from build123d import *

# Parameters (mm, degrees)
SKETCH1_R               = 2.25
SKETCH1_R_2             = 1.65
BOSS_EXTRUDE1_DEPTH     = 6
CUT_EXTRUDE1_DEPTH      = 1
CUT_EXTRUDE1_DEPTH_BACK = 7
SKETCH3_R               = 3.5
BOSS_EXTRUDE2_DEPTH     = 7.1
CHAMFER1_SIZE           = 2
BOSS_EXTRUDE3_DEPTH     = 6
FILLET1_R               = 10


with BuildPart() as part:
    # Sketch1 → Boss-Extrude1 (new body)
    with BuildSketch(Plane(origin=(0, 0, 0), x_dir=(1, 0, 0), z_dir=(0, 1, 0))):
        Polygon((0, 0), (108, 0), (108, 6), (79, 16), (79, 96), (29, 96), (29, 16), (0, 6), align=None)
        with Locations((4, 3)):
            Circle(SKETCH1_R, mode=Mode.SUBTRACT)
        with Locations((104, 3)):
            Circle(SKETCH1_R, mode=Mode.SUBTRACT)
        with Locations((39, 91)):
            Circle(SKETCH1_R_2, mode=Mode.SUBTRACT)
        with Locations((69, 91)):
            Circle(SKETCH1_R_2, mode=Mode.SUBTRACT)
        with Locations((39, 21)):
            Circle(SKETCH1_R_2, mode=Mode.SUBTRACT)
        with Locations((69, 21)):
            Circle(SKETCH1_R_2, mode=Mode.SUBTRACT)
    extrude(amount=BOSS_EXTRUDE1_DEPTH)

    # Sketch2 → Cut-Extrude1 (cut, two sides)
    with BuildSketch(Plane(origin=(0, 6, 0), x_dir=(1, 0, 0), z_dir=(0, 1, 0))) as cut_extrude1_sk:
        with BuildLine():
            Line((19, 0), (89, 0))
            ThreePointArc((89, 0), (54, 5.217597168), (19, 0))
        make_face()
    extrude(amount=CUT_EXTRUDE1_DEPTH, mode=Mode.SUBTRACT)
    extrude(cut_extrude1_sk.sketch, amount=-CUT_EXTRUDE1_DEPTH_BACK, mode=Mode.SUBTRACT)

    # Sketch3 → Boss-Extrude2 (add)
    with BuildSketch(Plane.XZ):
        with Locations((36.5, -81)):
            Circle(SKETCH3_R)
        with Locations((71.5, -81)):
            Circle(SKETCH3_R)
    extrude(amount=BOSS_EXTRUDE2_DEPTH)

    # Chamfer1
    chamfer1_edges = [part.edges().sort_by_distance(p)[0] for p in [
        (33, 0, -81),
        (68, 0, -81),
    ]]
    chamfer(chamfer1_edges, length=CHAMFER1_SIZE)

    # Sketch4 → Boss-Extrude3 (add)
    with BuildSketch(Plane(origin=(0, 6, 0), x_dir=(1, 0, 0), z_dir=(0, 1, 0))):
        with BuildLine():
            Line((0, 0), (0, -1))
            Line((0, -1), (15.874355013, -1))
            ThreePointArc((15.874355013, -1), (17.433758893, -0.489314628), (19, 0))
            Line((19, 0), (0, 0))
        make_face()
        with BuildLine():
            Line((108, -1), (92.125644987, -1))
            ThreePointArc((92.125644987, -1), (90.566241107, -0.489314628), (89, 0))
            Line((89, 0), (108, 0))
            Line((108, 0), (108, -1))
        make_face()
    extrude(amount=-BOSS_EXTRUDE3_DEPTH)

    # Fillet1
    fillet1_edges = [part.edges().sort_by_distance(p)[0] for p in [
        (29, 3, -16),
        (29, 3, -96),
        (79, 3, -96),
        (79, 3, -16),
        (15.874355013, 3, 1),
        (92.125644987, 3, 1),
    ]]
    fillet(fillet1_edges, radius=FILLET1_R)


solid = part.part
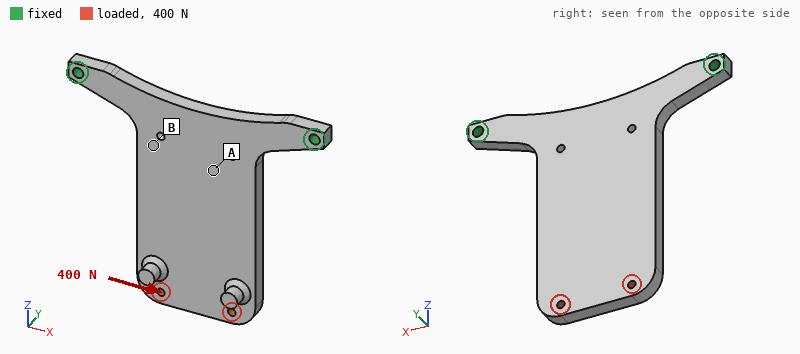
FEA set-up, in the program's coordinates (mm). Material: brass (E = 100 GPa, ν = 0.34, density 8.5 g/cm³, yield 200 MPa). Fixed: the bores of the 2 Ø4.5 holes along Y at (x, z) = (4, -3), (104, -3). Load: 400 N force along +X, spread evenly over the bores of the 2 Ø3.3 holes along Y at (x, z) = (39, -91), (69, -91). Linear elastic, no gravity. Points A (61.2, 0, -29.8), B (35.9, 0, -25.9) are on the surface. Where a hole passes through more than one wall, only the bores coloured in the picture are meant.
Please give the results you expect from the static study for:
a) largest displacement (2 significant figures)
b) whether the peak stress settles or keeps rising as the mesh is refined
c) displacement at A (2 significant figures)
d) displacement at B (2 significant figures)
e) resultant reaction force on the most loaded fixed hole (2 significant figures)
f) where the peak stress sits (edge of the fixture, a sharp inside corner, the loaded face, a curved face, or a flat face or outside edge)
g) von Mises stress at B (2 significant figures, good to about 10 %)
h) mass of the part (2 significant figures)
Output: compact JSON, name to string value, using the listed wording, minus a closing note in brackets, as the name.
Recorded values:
{"largest displacement": "50 µm", "whether the peak stress settles or keeps rising as the mesh is refined": "keeps rising", "displacement at A": "8.2 µm", "displacement at B": "10 µm", "resultant reaction force on the most loaded fixed hole": "460 N", "where the peak stress sits": "edge of the fixture", "von Mises stress at B": "8.6 MPa", "mass of the part": "270 g"}
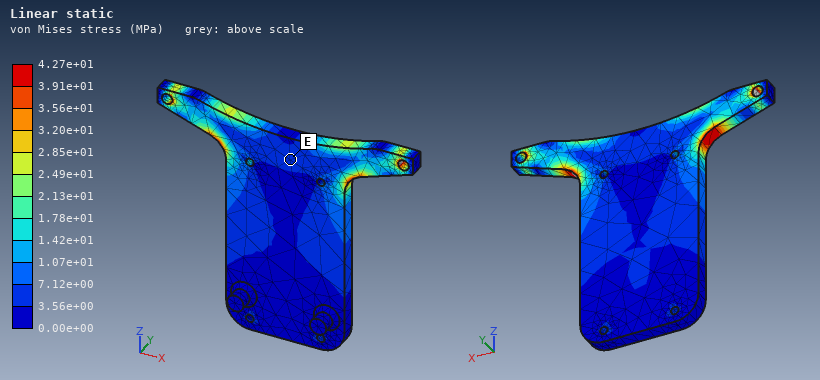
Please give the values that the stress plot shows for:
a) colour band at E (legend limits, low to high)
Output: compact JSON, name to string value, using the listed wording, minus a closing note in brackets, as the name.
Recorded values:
{"colour band at E": "3.56e+00 to 7.12e+00 MPa"}
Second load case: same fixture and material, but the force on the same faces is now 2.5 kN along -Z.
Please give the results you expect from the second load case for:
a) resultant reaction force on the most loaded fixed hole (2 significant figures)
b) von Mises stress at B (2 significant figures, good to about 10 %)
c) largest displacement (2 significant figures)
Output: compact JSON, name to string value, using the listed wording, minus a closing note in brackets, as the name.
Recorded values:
{"resultant reaction force on the most loaded fixed hole": "2.2 kN", "von Mises stress at B": "19 MPa", "largest displacement": "48 µm"}
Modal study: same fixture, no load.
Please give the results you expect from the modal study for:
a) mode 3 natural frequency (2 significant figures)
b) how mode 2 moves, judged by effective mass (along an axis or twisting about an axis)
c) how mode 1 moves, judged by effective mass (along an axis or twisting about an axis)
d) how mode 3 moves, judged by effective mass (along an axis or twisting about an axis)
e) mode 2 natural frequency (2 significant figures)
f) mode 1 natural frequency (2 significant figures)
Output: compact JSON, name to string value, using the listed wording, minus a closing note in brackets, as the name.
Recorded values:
{"mode 3 natural frequency": "1400 Hz", "how mode 2 moves, judged by effective mass": "twisting about Z", "how mode 1 moves, judged by effective mass": "along Y", "how mode 3 moves, judged by effective mass": "along Y", "mode 2 natural frequency": "1300 Hz", "mode 1 natural frequency": "210 Hz"}
